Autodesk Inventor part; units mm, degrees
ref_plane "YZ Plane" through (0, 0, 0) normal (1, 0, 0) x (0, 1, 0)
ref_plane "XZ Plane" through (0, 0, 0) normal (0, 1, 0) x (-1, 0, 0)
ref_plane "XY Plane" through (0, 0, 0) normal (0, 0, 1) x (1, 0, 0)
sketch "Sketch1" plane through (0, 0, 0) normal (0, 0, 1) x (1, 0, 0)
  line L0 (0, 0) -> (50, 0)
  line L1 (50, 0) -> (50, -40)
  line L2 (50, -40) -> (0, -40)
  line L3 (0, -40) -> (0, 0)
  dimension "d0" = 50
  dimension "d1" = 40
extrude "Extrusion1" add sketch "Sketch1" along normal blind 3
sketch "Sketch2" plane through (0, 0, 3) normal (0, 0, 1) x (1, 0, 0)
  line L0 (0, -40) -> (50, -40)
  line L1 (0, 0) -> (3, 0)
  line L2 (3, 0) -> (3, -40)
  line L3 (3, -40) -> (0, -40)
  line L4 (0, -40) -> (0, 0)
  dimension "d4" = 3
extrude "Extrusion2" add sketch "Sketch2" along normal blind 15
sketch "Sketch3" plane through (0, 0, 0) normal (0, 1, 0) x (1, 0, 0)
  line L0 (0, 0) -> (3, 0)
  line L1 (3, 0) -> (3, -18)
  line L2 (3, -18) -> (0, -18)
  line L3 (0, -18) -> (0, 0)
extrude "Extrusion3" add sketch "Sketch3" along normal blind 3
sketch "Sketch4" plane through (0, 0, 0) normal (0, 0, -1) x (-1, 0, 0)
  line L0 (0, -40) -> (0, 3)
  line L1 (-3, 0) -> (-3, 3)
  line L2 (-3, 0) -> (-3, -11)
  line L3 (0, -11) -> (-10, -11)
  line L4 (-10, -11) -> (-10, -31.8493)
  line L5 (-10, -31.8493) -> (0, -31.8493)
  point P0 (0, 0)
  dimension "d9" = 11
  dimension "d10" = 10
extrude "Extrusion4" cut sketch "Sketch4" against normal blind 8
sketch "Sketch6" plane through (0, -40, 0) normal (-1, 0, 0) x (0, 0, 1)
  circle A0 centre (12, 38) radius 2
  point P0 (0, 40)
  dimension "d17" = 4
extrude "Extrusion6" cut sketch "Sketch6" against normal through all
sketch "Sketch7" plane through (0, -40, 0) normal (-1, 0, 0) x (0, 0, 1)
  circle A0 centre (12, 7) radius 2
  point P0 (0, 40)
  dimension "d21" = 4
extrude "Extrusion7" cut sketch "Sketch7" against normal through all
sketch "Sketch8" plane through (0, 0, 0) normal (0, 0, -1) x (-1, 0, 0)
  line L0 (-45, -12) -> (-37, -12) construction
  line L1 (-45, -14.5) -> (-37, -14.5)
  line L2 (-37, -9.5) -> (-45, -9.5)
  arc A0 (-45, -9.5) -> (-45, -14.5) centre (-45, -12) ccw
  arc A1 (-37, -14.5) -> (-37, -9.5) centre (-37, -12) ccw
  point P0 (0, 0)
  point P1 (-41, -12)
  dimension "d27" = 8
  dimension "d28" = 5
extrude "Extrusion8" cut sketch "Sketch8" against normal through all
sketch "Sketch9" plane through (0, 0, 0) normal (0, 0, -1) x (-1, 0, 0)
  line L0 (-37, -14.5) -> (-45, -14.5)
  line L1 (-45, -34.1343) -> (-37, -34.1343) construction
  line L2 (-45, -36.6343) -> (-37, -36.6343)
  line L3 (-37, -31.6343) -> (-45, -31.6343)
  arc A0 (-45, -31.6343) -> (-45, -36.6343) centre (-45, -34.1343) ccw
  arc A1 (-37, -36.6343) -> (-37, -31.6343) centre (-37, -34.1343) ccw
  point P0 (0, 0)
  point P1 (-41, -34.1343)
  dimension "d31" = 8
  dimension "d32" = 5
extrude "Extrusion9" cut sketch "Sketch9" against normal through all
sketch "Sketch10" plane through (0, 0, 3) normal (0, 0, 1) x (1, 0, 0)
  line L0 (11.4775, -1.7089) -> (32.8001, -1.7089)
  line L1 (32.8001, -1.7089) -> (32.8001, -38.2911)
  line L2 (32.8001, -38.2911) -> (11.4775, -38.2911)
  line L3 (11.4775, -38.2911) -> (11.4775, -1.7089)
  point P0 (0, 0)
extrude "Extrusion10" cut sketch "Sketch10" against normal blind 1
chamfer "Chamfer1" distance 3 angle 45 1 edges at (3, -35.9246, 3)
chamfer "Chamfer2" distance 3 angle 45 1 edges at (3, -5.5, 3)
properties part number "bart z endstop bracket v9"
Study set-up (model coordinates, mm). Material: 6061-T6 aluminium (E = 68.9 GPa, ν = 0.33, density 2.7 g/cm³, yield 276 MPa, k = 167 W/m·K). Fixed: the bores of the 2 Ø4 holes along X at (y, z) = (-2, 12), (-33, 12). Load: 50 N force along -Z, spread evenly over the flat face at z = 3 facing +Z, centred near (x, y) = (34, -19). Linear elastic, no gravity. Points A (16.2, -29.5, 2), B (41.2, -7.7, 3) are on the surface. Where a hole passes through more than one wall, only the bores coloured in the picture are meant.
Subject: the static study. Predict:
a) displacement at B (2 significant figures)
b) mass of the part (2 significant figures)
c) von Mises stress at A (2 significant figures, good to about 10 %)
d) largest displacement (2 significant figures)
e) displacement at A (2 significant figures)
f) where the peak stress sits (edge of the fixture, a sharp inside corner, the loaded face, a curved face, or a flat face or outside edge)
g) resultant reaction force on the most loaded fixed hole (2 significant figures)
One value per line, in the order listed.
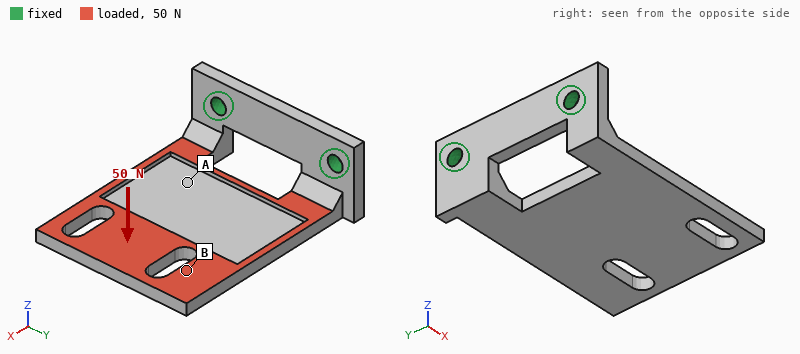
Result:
0.39 mm
16 g
23 MPa
0.53 mm
0.090 mm
a flat face or outside edge
26 N
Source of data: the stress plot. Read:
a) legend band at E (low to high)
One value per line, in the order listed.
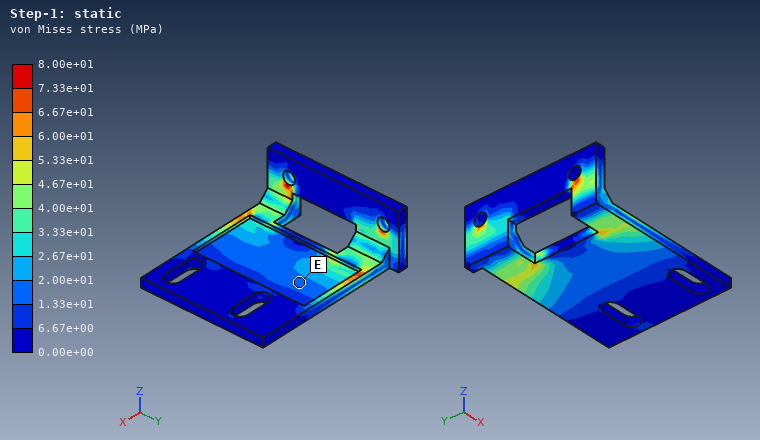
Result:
1.33e+01 to 2.00e+01 MPa
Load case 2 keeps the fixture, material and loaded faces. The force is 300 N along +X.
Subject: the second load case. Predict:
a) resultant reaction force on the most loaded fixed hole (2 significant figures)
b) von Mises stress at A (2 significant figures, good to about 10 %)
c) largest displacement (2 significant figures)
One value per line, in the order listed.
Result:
150 N
17 MPa
57 µm
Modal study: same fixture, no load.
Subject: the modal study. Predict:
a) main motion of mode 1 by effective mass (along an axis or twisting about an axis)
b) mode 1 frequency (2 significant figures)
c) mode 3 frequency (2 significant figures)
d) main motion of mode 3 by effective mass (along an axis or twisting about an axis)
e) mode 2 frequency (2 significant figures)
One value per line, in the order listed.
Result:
along Z
660 Hz
3300 Hz
along Y
2000 Hz
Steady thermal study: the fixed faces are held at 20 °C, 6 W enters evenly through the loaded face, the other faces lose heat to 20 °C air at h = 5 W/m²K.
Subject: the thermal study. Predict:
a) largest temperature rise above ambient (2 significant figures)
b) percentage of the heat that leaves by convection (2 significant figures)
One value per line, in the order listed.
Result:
20 K
4.1 %
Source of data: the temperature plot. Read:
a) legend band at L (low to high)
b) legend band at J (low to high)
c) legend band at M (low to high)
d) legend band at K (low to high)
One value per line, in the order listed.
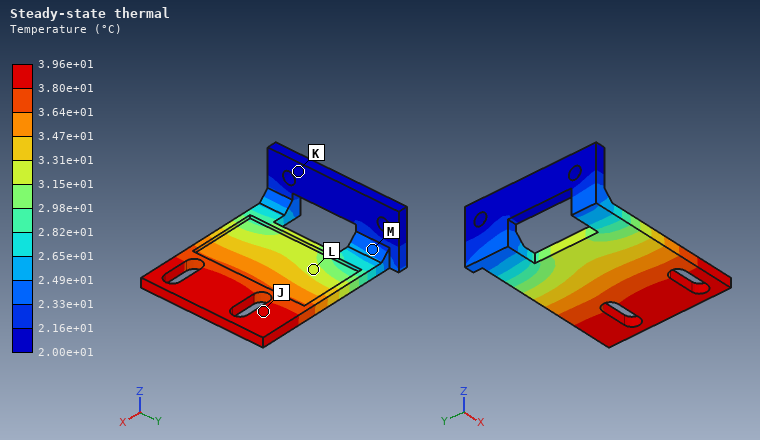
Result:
3.15e+01 to 3.31e+01 °C
3.80e+01 to 3.96e+01 °C
2.33e+01 to 2.49e+01 °C
2.00e+01 to 2.16e+01 °C
